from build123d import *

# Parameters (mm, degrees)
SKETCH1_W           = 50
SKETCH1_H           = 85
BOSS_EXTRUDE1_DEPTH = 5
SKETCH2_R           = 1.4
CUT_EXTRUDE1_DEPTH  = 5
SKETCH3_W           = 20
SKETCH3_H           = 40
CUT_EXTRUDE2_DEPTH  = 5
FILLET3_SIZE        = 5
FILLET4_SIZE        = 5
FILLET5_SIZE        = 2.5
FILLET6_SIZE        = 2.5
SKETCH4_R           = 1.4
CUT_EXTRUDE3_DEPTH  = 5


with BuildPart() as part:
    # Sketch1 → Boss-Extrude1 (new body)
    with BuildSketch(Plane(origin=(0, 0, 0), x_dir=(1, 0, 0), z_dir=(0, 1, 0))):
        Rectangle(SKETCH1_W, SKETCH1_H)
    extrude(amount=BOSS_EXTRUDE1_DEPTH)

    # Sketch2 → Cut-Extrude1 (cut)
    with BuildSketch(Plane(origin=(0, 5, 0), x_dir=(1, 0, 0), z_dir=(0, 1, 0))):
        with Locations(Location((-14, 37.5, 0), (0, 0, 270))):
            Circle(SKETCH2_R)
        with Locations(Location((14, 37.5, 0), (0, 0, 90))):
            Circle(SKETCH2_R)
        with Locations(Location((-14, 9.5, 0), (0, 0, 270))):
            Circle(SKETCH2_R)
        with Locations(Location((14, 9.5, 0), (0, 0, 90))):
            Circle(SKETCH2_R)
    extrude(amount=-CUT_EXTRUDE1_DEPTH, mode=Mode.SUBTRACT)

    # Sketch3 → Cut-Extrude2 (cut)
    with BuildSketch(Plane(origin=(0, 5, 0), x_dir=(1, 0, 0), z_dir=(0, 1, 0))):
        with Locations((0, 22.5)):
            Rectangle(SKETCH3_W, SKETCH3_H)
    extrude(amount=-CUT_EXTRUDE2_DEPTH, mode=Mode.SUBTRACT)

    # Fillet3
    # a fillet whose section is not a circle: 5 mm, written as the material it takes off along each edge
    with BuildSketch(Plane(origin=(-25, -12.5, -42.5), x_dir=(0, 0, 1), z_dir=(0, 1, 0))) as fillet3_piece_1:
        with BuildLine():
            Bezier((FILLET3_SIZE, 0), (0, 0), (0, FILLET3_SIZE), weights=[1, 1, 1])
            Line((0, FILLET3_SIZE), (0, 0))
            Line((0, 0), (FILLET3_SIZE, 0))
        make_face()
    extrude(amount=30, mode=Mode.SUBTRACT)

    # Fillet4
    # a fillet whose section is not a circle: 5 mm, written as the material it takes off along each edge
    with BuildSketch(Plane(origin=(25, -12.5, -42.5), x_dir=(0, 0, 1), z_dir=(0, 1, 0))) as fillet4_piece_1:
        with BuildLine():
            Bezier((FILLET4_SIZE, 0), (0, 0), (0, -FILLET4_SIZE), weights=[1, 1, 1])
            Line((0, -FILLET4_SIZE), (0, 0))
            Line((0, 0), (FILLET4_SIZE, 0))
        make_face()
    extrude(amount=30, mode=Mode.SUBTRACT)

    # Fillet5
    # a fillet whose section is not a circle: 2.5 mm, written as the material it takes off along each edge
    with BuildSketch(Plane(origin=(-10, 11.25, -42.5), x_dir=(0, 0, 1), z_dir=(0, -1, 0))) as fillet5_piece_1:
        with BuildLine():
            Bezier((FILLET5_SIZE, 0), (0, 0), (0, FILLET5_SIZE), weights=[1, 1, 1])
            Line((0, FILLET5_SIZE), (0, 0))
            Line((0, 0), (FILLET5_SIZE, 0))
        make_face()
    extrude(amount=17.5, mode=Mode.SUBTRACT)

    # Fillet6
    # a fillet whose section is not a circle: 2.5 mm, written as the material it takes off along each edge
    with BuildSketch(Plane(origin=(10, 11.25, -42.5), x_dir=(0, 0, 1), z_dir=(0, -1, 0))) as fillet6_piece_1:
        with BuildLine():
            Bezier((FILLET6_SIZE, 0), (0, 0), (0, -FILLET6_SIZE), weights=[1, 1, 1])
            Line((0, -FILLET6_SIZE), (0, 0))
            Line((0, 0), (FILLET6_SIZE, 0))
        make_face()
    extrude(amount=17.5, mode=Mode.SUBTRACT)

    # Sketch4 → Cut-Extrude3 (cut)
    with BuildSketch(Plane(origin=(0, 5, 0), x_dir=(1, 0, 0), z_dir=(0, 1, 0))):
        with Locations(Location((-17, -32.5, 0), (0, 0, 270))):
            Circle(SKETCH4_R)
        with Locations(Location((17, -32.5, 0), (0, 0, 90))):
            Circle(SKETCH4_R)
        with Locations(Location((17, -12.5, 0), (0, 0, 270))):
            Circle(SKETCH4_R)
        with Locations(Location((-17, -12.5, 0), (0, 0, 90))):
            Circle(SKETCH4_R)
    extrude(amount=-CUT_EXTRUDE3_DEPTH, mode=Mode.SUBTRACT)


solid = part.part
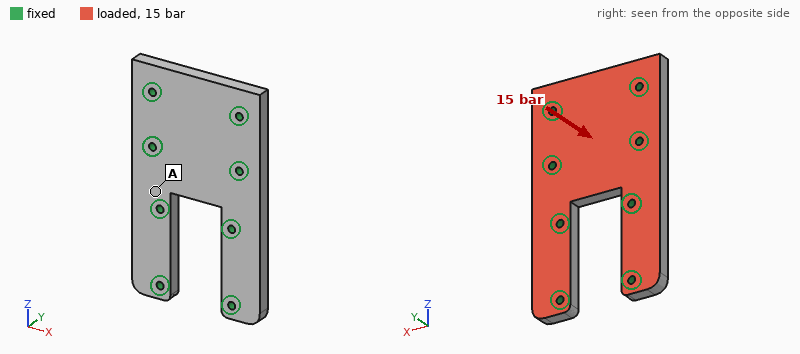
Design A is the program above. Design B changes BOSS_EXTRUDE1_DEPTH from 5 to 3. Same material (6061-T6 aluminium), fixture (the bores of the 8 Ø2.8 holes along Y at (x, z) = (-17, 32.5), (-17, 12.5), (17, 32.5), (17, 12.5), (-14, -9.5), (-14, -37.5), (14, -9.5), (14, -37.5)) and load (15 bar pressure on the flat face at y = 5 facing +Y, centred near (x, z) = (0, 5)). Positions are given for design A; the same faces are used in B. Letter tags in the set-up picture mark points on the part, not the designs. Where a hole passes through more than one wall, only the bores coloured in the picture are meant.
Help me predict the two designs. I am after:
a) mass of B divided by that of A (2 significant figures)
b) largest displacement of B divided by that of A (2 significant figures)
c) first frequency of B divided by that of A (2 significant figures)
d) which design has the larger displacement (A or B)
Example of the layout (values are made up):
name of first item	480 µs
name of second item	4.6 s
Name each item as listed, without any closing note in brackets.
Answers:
mass of B divided by that of A	0.60
largest displacement of B divided by that of A	3.7
first frequency of B divided by that of A	0.68
which design has the larger displacement	B
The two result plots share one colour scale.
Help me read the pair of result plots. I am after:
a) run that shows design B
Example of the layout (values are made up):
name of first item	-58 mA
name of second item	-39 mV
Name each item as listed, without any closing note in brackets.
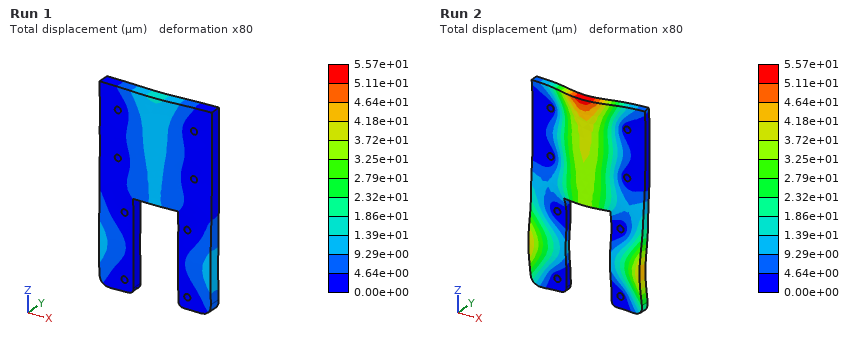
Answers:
run that shows design B	Run 2
